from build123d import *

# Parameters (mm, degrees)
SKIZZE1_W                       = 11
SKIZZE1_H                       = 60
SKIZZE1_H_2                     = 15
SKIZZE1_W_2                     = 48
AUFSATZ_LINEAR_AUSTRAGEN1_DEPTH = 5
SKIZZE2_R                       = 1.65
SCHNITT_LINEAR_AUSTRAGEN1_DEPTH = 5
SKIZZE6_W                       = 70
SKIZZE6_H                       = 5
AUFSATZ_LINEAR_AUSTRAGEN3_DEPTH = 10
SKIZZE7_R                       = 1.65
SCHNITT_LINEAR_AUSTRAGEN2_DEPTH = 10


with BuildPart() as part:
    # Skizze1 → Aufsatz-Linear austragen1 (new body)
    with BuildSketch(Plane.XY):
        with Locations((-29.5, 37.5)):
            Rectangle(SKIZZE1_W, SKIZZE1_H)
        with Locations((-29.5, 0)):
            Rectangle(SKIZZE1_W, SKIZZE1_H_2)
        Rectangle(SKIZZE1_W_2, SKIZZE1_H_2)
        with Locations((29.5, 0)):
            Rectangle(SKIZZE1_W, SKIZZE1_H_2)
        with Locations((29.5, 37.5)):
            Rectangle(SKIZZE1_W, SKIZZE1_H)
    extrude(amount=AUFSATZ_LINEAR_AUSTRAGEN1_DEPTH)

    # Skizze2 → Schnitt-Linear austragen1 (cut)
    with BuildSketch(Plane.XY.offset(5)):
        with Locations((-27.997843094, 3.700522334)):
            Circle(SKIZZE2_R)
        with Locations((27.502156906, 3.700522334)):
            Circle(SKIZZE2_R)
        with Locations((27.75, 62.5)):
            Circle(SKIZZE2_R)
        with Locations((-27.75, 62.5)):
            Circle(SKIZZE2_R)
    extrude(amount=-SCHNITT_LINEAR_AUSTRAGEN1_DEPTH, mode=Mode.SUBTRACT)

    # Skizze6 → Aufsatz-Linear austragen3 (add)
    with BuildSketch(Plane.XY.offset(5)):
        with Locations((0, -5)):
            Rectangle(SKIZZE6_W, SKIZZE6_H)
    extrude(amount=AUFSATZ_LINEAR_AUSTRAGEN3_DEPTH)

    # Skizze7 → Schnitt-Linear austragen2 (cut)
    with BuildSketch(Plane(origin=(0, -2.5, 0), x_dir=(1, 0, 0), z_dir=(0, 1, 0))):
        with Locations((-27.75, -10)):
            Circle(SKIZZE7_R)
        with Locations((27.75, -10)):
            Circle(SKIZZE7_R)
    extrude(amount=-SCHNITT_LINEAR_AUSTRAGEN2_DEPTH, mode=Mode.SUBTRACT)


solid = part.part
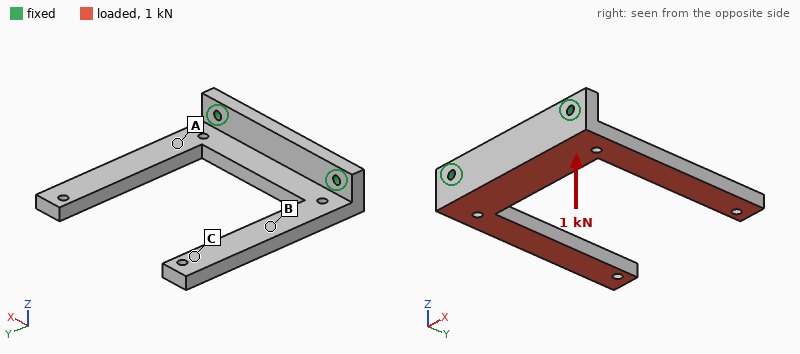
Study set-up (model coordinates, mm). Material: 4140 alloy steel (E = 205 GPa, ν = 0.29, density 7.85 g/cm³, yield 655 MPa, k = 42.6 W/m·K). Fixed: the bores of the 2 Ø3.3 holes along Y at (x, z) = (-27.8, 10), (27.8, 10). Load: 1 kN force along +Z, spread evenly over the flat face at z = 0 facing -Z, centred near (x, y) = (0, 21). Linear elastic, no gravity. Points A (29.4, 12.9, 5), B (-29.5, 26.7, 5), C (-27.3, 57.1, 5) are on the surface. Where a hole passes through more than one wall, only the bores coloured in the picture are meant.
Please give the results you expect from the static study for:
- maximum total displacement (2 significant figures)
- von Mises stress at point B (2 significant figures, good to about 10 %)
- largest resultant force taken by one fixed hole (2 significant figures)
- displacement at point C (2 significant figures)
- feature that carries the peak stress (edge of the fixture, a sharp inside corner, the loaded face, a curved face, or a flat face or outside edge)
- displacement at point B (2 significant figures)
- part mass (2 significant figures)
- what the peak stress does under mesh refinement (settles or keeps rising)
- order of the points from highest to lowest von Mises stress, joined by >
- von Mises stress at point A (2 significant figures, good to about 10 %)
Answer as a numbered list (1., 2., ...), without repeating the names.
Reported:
1. 0.75 mm
2. 83 MPa
3. 510 N
4. 0.60 mm
5. edge of the fixture
6. 0.22 mm
7. 120 g
8. keeps rising
9. A > B > C
10. 150 MPa
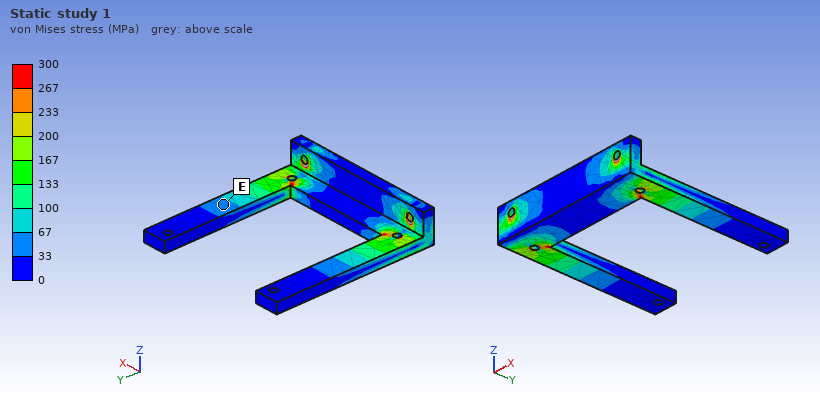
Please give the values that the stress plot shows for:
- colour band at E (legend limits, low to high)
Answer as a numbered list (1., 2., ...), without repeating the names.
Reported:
1. 33 to 67 MPa
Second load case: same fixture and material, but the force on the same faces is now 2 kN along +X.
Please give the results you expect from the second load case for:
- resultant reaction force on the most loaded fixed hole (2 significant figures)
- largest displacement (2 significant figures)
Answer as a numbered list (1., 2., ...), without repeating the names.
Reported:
1. 1.3 kN
2. 0.24 mm
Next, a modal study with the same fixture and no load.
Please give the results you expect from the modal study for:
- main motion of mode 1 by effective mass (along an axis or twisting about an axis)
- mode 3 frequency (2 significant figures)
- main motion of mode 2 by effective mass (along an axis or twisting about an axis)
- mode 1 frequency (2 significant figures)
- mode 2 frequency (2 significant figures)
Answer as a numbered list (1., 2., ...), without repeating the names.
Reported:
1. along Z
2. 1800 Hz
3. twisting about Y
4. 770 Hz
5. 800 Hz
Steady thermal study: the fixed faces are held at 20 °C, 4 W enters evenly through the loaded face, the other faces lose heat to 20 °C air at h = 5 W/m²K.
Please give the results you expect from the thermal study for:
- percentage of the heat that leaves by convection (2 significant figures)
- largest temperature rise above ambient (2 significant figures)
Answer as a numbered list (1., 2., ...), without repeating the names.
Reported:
1. 7.3 %
2. 21 K
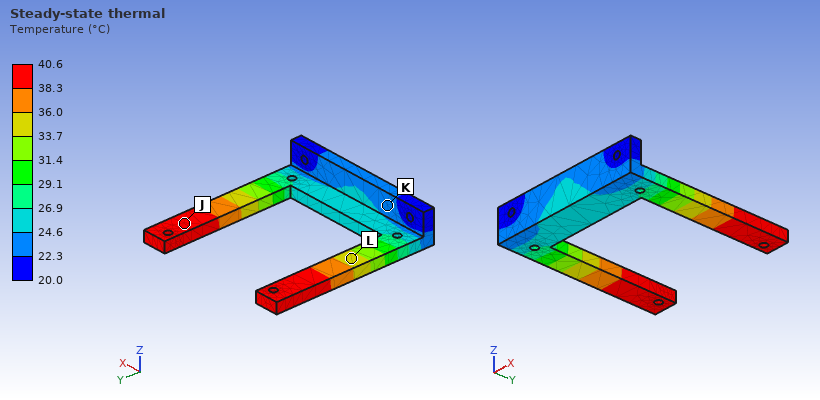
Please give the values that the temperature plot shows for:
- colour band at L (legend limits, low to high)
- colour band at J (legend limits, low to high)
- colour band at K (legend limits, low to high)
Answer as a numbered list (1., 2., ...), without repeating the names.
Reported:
1. 33.7 to 36.0 °C
2. 38.3 to 40.6 °C
3. 22.3 to 24.6 °C
